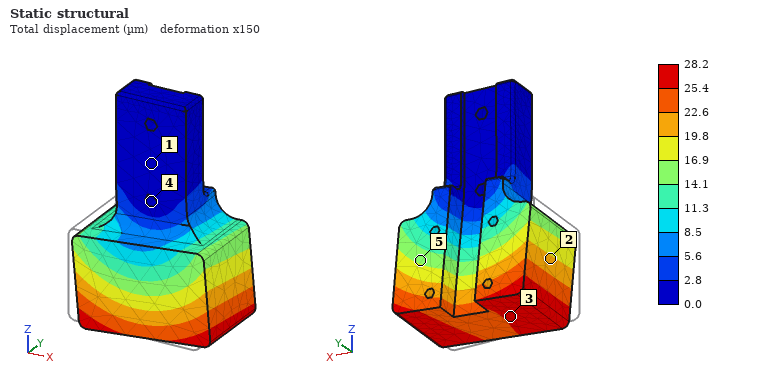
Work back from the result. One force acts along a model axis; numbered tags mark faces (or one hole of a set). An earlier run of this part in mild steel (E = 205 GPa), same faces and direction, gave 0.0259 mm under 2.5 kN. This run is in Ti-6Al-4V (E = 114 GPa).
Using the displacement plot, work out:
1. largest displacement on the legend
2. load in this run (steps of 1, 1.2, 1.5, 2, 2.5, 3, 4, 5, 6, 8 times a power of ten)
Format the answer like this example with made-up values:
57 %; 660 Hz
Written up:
28.2 µm; 1.5 kN
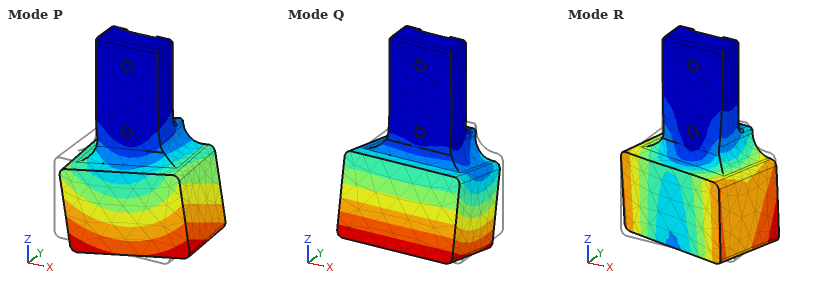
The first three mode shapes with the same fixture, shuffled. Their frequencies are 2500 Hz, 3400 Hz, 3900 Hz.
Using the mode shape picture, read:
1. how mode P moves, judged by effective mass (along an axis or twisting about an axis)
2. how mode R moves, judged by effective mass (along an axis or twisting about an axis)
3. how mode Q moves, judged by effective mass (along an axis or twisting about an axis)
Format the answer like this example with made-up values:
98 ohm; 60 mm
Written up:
along X; twisting about Z; along Y
